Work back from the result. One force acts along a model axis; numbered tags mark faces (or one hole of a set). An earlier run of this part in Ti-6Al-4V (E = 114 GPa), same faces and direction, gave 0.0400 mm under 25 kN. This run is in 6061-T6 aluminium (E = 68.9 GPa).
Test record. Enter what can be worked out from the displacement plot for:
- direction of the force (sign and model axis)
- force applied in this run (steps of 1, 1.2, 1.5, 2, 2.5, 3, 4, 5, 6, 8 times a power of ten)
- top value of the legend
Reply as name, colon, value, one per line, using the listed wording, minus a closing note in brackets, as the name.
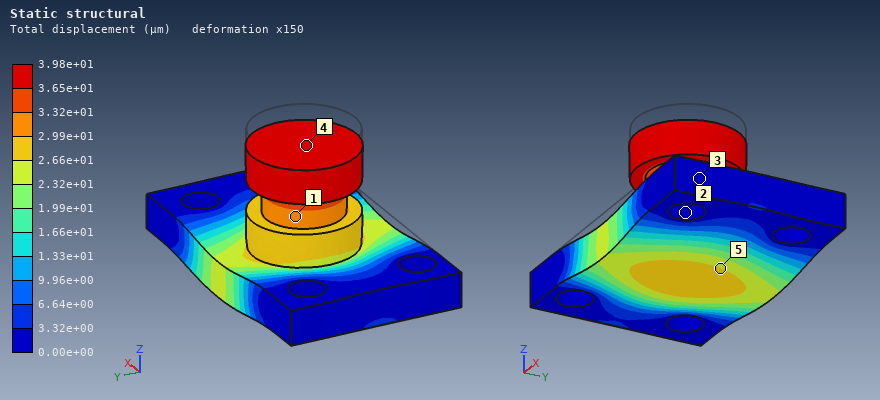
direction of the force: -Z
force applied in this run: 15 kN
top value of the legend: 3.98e+01 µm
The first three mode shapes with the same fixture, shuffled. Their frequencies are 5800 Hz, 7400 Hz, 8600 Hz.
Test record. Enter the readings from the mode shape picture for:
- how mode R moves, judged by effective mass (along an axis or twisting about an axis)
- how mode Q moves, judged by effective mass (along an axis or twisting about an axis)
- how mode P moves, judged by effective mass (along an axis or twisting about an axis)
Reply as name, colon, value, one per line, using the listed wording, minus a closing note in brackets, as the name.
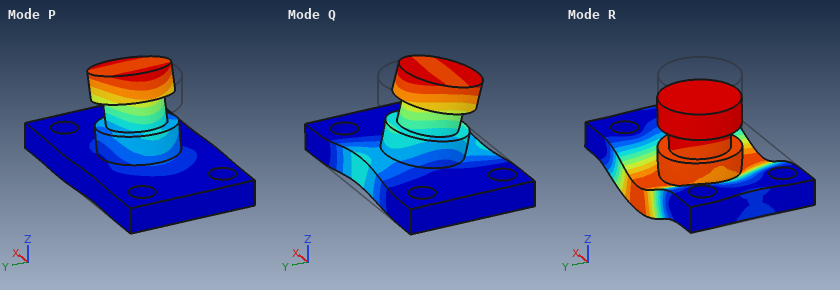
how mode R moves, judged by effective mass: along Z
how mode Q moves, judged by effective mass: along Y
how mode P moves, judged by effective mass: along X
